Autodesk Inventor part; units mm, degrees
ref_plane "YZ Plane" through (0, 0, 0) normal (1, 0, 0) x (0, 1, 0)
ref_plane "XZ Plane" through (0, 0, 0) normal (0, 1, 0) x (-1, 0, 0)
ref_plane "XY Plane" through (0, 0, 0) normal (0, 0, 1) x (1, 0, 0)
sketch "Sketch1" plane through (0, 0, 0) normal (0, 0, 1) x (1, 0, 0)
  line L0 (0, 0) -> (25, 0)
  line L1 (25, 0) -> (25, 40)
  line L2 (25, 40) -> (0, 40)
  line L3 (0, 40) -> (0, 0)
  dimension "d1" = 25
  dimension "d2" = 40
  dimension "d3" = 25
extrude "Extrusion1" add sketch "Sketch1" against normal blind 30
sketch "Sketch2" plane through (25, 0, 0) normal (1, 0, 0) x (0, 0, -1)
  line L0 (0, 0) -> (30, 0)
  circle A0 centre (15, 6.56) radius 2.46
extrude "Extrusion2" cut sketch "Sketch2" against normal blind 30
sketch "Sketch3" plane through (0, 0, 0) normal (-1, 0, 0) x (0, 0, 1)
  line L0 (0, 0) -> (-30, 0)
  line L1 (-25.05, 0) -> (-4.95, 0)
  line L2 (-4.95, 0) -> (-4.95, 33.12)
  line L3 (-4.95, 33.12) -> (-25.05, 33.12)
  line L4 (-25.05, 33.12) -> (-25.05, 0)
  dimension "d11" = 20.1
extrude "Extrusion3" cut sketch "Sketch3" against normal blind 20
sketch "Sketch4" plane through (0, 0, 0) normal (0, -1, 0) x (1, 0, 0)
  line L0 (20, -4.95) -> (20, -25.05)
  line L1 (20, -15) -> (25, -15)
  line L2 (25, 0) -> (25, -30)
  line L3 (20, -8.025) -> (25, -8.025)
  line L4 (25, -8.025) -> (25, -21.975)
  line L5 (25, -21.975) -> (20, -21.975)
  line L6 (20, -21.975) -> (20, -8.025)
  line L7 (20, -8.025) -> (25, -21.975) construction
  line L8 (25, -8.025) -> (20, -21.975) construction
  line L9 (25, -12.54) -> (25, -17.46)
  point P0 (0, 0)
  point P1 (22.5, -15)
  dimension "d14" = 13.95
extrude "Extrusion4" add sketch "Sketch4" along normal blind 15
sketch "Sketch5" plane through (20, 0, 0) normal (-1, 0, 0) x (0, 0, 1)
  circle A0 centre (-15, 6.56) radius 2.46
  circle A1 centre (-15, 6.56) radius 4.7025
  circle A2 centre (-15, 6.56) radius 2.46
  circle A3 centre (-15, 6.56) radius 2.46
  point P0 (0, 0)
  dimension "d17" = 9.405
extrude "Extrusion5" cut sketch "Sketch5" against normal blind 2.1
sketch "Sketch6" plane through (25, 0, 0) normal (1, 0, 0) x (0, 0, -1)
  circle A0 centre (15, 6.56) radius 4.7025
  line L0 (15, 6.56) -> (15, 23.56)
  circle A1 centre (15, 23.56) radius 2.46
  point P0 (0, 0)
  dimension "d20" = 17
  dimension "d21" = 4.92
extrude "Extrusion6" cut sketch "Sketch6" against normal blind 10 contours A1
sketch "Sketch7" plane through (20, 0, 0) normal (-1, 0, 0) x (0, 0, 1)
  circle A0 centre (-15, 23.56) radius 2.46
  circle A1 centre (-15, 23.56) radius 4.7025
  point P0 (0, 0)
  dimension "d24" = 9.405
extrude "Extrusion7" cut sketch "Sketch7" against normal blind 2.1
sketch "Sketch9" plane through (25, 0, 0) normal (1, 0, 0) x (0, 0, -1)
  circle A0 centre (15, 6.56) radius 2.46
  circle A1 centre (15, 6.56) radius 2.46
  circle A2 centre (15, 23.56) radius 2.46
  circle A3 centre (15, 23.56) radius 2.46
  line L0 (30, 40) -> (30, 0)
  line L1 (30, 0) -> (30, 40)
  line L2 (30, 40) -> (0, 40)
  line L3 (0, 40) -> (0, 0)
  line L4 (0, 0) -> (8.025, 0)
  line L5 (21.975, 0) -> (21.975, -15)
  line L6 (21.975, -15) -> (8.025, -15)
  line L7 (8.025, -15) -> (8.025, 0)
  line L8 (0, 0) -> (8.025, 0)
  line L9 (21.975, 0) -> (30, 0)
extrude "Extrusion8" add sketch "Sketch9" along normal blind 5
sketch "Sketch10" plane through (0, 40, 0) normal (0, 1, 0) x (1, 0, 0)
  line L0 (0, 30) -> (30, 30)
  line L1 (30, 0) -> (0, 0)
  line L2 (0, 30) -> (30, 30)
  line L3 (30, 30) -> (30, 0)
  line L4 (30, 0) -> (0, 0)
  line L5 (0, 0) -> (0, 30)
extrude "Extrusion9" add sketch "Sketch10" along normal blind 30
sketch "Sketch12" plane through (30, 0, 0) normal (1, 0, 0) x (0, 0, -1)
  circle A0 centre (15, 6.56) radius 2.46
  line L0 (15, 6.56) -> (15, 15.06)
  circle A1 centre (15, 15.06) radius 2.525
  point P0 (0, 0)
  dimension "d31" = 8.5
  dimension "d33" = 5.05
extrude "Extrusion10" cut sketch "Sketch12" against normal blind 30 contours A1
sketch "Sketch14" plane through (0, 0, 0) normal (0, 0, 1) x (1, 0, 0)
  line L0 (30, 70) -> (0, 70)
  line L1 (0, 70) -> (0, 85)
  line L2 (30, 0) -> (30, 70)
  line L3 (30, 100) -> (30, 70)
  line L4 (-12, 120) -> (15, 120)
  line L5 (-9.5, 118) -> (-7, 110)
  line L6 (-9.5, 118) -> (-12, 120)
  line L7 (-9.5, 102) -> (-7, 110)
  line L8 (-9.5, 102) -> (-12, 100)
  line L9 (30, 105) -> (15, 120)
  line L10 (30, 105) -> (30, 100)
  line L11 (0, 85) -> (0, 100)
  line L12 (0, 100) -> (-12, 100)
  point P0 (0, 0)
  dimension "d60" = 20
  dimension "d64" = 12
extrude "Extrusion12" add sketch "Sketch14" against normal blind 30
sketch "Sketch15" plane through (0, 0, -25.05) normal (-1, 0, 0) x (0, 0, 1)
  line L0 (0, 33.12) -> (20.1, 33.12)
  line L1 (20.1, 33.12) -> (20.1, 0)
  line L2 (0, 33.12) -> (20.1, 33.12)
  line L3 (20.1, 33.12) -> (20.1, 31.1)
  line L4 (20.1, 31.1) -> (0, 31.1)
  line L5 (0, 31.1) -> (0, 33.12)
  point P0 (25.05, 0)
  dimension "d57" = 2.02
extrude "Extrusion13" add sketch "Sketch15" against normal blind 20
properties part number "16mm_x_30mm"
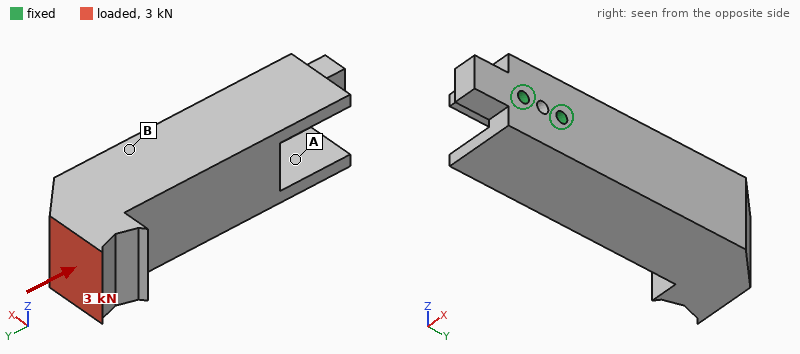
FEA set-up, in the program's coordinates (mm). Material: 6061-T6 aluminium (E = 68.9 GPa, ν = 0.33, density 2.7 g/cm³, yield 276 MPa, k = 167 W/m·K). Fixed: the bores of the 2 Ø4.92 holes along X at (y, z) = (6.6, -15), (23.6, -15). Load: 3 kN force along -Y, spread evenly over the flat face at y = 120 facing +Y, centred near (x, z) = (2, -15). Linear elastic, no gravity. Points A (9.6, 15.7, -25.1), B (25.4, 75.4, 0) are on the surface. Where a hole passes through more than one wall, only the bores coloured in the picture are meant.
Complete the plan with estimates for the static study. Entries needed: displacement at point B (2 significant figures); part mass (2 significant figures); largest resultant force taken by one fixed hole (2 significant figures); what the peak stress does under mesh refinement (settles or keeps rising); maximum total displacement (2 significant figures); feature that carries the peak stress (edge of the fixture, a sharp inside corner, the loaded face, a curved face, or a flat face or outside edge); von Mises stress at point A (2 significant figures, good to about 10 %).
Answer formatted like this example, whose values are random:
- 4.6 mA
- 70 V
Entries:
- 0.090 mm
- 270 g
- 3.4 kN
- keeps rising
- 0.21 mm
- edge of the fixture
- 22 MPa
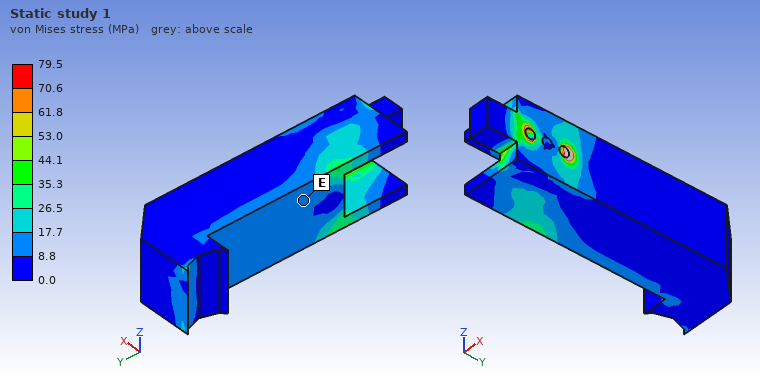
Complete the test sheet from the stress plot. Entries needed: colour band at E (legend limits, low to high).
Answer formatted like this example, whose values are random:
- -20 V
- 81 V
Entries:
- 8.8 to 17.7 MPa
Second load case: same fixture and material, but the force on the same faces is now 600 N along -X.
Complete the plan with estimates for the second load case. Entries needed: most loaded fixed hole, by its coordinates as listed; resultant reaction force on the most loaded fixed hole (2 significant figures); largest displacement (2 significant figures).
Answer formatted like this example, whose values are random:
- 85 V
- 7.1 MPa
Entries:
- (23.6, -15)
- 2.9 kN
- 0.17 mm
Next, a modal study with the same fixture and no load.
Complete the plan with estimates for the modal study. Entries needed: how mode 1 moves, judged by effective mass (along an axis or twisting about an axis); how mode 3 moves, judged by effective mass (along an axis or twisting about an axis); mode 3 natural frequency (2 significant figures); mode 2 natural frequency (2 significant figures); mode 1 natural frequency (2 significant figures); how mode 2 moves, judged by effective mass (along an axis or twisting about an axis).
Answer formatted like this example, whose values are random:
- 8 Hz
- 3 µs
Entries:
- along X
- twisting about Y
- 3300 Hz
- 1300 Hz
- 1100 Hz
- along Z
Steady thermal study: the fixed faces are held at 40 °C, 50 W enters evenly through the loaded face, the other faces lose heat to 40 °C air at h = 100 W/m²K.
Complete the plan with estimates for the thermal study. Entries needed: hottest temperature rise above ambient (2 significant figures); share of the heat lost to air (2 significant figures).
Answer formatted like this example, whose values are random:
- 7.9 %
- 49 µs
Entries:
- 34 K
- 44 %
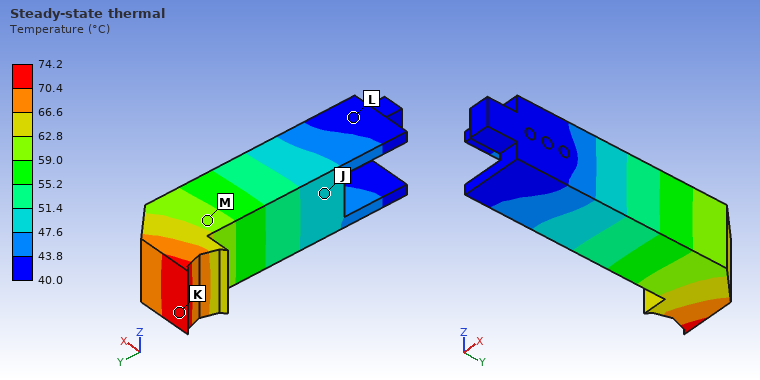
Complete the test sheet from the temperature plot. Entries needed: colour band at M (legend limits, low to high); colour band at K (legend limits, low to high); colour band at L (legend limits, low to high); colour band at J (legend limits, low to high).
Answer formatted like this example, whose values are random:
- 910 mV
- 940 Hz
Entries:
- 59.0 to 62.8 °C
- 70.4 to 74.2 °C
- 40.0 to 43.8 °C
- 47.6 to 51.4 °C
